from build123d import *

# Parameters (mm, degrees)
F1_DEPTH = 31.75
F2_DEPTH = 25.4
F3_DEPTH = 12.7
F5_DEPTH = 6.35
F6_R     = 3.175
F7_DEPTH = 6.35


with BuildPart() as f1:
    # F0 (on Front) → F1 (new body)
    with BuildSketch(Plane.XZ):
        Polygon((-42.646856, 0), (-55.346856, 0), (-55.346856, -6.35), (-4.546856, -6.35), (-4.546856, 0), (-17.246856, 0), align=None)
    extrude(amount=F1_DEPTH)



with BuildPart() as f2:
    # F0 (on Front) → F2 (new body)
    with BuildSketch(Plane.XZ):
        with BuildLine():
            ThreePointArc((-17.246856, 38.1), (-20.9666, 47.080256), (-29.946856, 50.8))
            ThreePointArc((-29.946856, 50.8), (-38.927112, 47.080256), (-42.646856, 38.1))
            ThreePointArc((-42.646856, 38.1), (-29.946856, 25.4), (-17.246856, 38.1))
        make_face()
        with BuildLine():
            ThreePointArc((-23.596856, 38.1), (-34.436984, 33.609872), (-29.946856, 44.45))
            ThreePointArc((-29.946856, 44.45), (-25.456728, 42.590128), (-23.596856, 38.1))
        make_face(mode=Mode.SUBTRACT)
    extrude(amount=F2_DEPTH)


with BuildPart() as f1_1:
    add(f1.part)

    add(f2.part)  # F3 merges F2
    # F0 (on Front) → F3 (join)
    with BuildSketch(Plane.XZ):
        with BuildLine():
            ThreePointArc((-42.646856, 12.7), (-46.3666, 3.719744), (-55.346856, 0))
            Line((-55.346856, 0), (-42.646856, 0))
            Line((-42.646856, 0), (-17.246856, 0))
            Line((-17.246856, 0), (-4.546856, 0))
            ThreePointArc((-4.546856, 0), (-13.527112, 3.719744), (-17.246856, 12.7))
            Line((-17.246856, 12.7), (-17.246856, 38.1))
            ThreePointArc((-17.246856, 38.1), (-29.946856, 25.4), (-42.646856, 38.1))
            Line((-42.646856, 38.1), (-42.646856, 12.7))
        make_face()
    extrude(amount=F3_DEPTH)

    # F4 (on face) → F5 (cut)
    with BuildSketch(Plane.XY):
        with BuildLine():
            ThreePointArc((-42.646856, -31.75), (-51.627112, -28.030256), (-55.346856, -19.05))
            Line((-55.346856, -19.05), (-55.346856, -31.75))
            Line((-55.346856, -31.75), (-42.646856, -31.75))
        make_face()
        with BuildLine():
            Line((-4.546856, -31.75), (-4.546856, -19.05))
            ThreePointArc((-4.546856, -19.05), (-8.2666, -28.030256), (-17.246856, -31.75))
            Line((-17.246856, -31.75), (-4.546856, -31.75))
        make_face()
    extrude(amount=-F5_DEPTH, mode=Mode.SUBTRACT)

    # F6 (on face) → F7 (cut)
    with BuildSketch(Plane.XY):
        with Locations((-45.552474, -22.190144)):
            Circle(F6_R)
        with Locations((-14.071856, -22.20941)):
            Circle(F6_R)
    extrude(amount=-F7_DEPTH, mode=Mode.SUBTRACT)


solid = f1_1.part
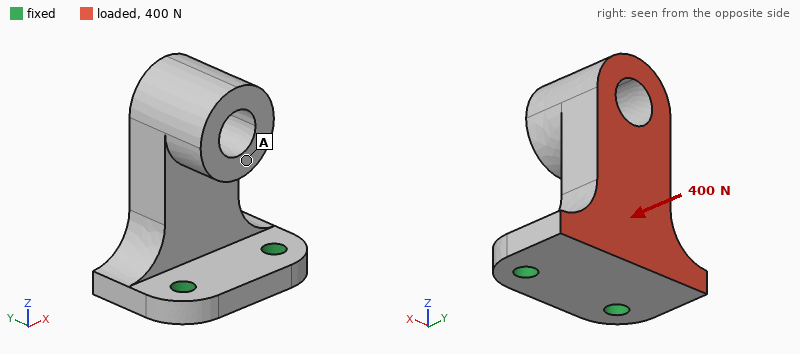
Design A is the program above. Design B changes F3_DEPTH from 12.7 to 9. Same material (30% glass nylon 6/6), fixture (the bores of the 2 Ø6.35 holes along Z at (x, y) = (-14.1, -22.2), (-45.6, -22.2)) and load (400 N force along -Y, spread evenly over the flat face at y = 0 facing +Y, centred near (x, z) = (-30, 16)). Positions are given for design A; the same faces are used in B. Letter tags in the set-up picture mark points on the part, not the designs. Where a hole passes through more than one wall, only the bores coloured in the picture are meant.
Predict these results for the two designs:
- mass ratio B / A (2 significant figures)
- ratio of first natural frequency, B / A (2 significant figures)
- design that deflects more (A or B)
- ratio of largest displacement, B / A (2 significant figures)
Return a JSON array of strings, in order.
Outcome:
["0.90", "0.83", "B", "1.5"]
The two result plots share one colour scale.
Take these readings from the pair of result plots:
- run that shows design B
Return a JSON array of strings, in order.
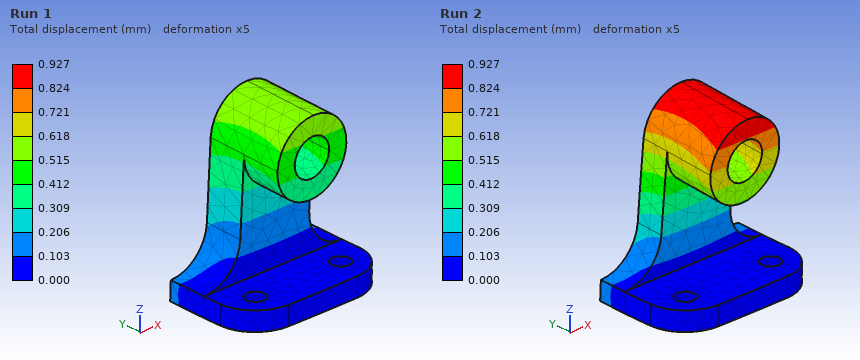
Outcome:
["Run 2"]
